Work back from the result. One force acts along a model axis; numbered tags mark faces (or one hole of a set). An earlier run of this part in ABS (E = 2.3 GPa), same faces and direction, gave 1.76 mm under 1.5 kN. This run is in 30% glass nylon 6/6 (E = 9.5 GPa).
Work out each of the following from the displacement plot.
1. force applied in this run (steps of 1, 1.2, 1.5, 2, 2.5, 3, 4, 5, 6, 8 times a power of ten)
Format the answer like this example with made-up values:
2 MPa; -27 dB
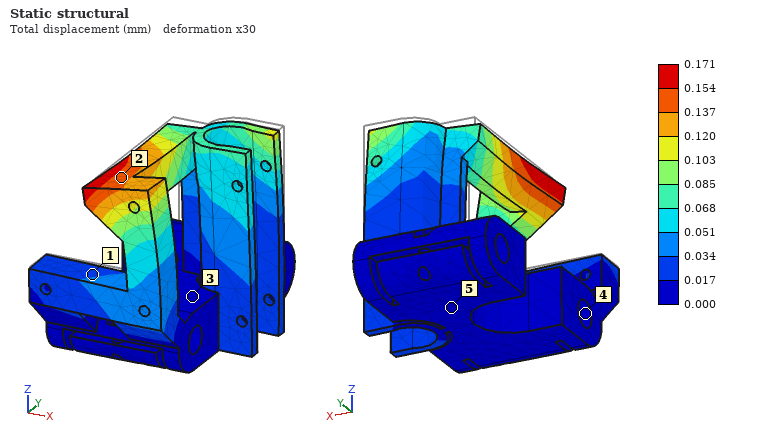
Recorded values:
600 N
